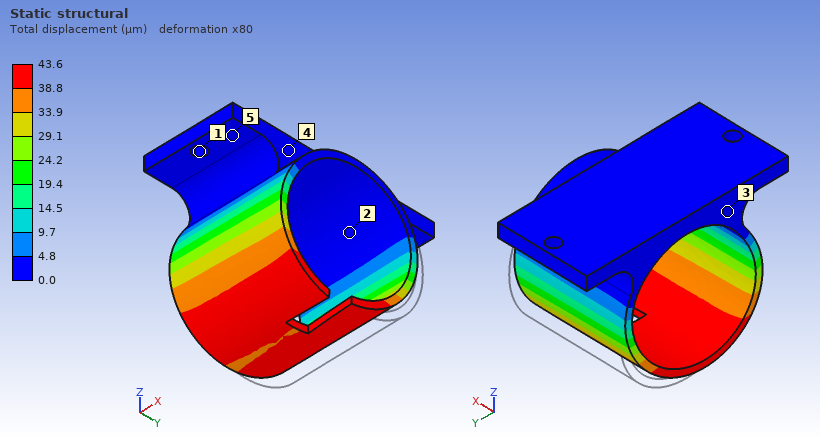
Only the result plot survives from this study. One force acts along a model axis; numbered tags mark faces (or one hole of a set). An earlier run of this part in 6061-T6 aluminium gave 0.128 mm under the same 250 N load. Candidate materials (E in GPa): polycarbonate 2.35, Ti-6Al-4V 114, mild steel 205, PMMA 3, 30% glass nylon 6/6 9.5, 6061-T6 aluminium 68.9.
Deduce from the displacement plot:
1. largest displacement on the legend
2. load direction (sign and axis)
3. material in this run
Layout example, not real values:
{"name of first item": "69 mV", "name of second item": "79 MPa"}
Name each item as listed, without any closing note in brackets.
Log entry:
{"largest displacement on the legend": "43.6 µm", "load direction": "-Y", "material in this run": "mild steel"}
